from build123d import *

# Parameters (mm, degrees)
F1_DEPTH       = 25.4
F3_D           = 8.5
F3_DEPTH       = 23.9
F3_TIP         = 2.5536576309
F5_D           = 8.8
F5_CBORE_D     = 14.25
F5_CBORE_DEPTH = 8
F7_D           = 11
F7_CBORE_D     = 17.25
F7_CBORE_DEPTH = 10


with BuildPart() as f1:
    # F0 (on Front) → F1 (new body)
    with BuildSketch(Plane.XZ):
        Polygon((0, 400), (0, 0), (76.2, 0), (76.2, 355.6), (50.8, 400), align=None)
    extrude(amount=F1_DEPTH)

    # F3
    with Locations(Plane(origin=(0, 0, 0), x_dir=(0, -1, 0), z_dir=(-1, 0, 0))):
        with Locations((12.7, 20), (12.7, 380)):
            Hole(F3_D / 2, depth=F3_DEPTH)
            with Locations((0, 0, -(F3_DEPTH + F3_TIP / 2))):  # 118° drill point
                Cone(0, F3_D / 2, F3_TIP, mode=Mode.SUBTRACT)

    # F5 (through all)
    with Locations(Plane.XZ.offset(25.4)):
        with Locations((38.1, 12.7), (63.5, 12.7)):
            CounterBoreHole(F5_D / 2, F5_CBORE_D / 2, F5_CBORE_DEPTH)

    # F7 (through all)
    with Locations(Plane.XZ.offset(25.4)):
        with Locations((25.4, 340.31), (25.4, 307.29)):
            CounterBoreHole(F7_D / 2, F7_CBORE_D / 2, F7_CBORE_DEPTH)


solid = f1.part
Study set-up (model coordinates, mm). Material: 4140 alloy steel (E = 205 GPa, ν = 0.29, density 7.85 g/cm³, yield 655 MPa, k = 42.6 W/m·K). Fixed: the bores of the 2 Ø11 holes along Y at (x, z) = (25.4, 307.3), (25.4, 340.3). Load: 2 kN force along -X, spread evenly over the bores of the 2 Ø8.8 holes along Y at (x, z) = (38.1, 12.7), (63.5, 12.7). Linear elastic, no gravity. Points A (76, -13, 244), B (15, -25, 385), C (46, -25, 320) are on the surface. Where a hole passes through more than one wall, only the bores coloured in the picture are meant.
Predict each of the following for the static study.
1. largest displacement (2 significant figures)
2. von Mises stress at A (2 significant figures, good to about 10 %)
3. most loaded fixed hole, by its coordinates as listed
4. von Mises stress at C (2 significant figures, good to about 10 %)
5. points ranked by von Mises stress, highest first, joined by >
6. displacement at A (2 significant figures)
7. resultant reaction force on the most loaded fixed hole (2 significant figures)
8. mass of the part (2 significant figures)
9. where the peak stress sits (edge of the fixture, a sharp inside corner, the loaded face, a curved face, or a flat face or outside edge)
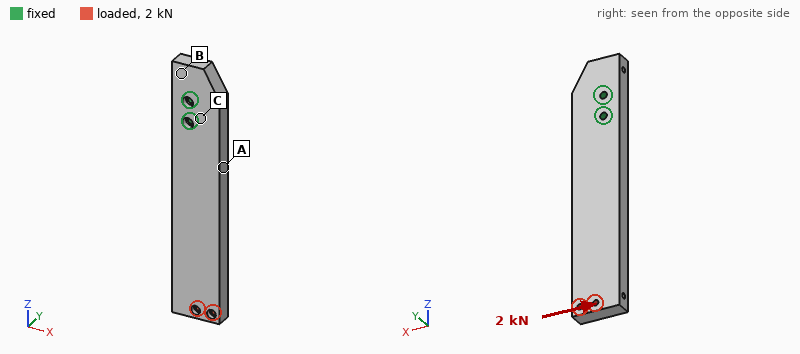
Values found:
0.16 mm
19 MPa
(25.4, 307.3)
11 MPa
A > C > B
0.027 mm
15 kN
5.8 kg
edge of the fixture
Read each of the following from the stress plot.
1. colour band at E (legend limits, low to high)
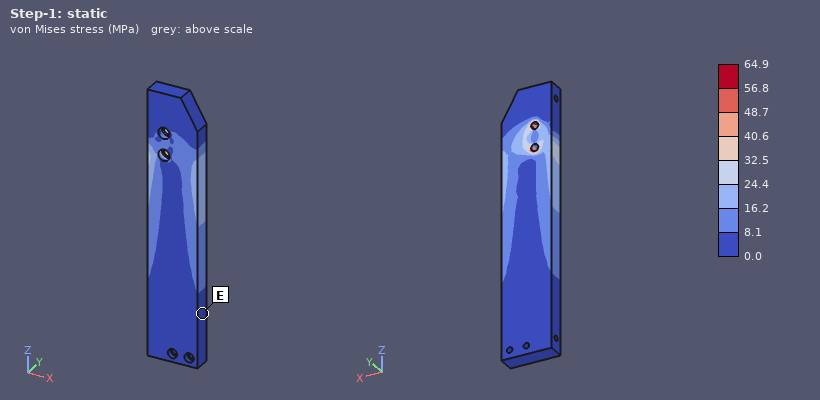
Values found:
0.0 to 8.1 MPa
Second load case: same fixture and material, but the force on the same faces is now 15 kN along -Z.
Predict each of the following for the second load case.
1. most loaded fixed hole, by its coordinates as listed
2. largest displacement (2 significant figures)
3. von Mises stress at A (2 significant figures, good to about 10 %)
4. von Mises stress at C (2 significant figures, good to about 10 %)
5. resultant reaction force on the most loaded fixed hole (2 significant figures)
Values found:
(25.4, 307.3)
0.17 mm
16 MPa
8.3 MPa
13 kN
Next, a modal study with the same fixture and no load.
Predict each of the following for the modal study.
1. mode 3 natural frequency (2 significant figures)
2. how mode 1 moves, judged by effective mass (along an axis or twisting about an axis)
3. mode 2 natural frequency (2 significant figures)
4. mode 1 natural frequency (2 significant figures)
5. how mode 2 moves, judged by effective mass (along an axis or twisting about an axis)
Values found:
1200 Hz
along Y
480 Hz
200 Hz
along X
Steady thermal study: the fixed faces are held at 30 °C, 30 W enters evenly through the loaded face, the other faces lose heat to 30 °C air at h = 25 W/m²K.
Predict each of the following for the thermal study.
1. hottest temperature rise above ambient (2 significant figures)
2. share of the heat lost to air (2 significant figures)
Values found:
46 K
86 %
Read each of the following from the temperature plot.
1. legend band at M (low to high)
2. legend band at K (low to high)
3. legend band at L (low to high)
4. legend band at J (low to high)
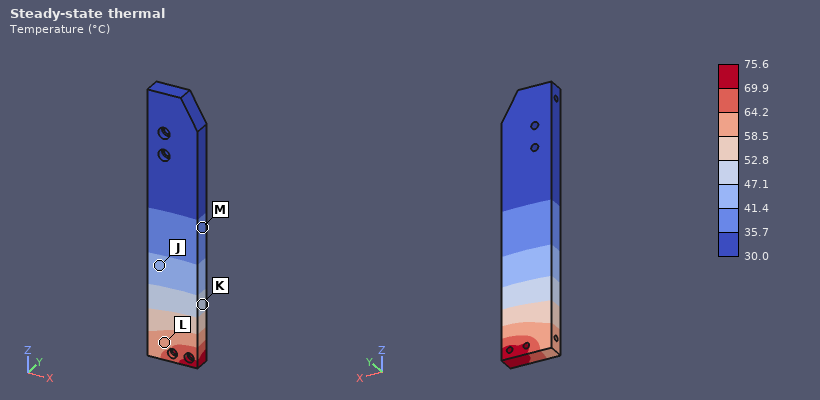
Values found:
35.7 to 41.4 °C
47.1 to 52.8 °C
58.5 to 64.2 °C
41.4 to 47.1 °C
